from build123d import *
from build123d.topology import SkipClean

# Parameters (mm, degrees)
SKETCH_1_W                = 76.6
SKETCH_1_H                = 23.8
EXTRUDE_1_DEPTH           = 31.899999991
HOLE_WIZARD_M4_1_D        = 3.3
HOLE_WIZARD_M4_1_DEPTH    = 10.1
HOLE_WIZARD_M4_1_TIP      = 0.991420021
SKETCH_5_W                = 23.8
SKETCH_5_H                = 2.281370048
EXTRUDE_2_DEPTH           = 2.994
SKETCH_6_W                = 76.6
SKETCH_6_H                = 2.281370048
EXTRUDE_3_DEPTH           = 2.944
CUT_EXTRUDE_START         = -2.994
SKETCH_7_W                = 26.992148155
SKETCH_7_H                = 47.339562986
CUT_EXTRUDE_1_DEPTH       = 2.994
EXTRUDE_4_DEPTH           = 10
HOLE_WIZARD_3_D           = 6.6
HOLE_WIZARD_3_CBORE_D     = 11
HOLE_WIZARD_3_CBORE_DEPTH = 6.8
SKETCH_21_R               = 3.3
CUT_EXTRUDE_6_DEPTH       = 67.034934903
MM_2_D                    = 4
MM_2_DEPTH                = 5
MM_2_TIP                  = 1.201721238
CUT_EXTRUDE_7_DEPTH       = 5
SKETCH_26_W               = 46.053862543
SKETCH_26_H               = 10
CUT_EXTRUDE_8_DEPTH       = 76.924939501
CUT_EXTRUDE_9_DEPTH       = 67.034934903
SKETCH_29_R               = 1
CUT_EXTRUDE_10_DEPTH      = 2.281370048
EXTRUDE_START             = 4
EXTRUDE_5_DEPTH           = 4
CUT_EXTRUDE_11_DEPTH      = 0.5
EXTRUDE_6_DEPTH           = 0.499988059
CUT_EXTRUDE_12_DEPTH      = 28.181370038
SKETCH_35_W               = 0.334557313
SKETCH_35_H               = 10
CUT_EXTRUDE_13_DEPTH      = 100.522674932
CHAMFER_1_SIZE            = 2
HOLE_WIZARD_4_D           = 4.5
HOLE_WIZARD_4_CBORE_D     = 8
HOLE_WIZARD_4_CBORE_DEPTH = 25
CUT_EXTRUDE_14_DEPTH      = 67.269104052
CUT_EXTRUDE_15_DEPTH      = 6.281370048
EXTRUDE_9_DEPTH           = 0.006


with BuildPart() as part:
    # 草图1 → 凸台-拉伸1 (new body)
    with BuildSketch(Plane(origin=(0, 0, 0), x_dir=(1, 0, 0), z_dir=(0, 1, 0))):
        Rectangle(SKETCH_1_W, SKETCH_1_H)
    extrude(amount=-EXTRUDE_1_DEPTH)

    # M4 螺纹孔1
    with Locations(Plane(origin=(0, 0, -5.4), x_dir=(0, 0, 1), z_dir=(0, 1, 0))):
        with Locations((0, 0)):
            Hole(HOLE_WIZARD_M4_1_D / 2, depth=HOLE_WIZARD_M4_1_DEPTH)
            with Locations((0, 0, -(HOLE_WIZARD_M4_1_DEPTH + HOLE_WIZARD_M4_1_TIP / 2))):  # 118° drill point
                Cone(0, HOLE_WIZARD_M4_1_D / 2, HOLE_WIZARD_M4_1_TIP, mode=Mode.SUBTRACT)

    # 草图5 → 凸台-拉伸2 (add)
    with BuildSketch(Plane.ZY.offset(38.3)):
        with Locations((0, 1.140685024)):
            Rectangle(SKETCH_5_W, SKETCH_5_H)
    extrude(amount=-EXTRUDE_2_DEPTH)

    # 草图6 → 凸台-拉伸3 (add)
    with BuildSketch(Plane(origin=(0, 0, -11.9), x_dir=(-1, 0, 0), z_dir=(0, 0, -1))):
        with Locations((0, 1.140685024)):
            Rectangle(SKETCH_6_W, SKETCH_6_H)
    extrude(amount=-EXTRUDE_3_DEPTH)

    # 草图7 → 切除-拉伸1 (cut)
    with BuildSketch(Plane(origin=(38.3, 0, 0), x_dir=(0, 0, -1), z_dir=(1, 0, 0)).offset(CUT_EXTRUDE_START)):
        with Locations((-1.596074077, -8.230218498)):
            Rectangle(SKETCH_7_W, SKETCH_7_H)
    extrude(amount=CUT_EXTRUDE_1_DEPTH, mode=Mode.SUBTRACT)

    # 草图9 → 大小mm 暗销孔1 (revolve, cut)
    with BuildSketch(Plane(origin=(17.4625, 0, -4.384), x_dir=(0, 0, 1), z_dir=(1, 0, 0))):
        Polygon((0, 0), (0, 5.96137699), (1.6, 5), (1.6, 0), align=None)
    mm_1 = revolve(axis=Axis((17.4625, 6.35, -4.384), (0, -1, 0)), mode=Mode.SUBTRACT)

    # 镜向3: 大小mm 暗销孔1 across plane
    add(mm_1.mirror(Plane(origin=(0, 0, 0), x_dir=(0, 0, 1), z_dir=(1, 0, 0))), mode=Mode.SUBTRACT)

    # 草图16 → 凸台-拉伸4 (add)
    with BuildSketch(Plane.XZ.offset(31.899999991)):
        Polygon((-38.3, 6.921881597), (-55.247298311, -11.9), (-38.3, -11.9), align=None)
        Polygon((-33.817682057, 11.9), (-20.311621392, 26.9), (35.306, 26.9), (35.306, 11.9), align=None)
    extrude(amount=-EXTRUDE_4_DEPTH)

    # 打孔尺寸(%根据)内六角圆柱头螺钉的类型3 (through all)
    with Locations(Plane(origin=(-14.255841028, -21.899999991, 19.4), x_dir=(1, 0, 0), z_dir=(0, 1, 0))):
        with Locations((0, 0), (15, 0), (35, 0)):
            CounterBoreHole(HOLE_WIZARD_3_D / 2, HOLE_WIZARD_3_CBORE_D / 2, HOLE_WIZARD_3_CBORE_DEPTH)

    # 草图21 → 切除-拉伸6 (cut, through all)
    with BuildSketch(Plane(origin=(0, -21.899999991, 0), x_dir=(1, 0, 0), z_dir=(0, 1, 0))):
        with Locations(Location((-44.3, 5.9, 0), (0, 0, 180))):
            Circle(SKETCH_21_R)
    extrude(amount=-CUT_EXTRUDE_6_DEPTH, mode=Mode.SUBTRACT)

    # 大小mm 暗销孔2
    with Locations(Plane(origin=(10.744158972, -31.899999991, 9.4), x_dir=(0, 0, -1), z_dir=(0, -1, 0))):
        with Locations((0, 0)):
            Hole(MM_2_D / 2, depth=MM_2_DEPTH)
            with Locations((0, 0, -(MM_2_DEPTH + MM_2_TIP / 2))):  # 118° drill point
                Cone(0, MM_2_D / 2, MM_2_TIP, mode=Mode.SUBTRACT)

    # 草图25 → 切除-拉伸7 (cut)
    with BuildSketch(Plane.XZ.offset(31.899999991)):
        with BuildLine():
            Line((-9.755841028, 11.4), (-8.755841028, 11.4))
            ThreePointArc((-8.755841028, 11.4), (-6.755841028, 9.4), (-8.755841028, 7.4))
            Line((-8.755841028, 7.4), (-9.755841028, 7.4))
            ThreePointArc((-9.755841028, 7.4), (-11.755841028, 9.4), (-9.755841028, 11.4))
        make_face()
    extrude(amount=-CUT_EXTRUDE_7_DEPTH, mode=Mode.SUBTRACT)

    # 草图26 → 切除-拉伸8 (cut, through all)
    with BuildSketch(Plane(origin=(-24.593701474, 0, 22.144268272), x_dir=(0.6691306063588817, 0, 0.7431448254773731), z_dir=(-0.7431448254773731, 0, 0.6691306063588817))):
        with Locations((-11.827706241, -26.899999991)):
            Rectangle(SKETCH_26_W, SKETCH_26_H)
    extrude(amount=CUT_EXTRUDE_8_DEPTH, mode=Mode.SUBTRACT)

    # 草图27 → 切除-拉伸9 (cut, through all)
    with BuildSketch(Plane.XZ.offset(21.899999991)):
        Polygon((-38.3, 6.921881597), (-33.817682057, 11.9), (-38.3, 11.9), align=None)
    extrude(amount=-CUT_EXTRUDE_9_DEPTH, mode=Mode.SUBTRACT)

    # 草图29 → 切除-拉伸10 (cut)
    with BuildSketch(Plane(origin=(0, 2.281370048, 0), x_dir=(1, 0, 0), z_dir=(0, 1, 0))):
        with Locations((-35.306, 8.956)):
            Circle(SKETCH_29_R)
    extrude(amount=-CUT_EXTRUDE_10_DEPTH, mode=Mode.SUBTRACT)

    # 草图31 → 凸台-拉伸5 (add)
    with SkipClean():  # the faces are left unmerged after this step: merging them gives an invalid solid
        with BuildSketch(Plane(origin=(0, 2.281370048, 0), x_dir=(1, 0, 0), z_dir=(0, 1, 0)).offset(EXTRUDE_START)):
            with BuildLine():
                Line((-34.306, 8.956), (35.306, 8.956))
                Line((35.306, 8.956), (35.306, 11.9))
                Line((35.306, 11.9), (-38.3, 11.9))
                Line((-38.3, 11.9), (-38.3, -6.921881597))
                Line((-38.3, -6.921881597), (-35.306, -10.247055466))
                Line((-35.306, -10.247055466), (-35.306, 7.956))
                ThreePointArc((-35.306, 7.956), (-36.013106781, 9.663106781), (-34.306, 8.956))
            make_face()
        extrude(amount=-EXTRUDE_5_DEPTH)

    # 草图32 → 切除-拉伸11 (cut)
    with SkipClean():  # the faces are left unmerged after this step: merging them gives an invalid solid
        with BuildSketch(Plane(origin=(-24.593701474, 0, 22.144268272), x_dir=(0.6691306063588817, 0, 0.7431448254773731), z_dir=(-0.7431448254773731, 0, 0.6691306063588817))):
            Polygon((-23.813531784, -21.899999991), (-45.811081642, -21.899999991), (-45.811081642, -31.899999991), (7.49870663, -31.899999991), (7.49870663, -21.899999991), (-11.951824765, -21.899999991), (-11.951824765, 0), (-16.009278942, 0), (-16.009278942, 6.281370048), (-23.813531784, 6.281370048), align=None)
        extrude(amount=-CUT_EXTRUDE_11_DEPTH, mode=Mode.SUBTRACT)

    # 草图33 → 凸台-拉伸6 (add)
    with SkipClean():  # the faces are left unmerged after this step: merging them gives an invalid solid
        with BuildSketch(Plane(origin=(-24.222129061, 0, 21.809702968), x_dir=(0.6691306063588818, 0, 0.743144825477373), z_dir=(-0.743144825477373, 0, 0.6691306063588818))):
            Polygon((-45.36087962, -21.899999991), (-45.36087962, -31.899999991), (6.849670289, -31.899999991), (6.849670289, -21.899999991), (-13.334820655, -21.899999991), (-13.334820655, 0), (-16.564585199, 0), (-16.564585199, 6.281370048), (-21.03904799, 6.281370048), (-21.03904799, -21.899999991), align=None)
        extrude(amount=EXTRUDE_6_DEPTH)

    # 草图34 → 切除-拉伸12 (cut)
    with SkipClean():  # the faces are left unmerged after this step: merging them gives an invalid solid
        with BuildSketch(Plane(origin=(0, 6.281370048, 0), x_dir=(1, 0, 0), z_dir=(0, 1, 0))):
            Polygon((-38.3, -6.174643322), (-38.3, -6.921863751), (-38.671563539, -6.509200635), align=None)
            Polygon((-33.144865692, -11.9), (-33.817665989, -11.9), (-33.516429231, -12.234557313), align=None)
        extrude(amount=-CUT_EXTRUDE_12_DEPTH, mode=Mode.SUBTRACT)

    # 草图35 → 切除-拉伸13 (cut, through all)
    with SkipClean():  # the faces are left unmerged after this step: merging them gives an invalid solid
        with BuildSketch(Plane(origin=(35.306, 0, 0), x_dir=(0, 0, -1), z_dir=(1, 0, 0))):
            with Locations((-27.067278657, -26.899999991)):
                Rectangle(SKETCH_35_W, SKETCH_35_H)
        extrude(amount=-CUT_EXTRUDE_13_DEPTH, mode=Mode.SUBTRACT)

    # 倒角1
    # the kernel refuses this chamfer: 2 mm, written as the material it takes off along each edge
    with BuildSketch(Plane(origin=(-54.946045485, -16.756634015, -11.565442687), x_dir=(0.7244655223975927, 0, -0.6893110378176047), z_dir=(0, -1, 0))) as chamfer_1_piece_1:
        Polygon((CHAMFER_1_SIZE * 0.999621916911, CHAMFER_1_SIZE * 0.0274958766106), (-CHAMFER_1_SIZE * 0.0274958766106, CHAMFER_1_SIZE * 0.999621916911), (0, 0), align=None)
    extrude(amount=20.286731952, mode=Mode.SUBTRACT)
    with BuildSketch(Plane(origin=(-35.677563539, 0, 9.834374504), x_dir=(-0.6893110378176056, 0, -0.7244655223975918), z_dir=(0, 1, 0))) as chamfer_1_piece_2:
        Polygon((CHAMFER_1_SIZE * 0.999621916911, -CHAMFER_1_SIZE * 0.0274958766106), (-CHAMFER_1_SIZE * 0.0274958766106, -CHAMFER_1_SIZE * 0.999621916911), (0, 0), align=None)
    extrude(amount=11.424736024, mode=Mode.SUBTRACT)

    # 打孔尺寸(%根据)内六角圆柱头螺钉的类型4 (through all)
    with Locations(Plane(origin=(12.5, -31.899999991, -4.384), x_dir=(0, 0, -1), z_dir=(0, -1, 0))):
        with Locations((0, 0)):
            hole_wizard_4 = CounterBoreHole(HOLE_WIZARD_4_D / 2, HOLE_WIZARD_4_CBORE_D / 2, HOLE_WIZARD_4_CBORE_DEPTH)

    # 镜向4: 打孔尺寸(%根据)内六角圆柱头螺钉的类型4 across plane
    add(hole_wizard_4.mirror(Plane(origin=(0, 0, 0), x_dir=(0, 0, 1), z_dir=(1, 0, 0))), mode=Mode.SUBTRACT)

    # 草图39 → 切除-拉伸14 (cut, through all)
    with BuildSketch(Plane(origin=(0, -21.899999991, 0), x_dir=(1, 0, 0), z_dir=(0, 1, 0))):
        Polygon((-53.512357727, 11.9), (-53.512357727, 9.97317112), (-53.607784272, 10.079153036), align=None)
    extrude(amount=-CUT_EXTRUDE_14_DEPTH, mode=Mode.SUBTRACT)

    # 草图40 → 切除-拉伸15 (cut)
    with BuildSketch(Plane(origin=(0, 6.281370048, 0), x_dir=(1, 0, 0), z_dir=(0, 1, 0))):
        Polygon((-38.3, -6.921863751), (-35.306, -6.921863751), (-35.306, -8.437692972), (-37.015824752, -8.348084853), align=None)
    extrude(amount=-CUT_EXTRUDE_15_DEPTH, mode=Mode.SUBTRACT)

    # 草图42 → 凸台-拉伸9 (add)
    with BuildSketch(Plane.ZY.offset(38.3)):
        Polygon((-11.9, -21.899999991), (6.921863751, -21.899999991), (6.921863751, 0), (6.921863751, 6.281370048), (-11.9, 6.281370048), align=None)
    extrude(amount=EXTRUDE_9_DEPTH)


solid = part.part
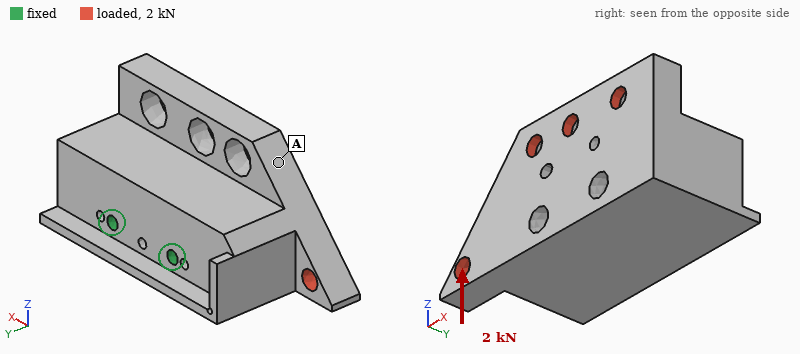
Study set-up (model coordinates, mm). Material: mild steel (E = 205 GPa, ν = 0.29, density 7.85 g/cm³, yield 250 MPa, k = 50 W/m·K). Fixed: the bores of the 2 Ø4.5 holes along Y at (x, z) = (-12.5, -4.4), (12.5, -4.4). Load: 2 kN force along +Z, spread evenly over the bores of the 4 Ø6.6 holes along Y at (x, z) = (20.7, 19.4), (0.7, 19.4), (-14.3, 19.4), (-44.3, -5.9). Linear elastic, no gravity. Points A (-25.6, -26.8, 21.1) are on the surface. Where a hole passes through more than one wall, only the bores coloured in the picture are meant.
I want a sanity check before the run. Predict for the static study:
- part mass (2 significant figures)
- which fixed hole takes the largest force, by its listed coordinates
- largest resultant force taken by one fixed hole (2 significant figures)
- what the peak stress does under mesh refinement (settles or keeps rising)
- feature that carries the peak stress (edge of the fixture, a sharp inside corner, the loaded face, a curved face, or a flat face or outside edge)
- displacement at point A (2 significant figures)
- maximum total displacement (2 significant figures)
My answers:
490 g
(-12.5, -4.4)
2.5 kN
keeps rising
edge of the fixture
27 µm
32 µm
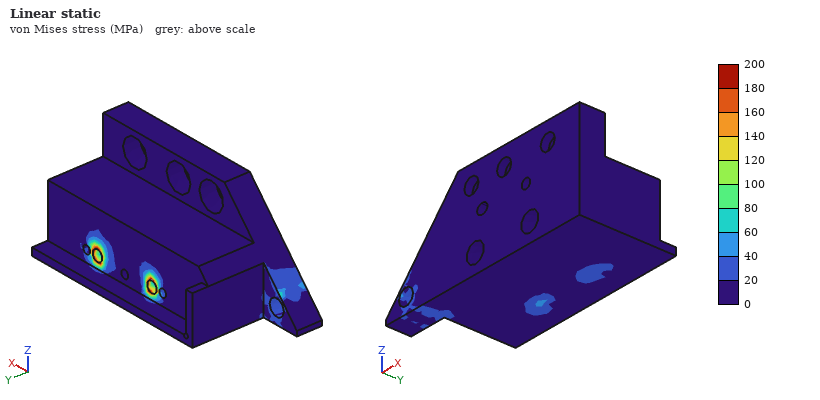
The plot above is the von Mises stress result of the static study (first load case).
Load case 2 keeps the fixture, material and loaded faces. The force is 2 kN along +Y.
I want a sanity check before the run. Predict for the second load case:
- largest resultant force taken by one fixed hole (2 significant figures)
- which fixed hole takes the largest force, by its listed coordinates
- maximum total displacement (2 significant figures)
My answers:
2.5 kN
(-12.5, -4.4)
16 µm
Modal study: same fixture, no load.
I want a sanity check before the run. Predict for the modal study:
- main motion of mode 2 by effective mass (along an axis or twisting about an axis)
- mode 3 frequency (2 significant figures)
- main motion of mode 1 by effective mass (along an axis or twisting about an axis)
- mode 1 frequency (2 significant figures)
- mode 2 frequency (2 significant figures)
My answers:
along X
6200 Hz
along Z
3100 Hz
5900 Hz
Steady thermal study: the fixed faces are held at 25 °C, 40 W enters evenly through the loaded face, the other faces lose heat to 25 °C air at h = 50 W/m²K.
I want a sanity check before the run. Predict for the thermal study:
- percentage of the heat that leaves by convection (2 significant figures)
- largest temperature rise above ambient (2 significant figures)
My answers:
32 %
74 K
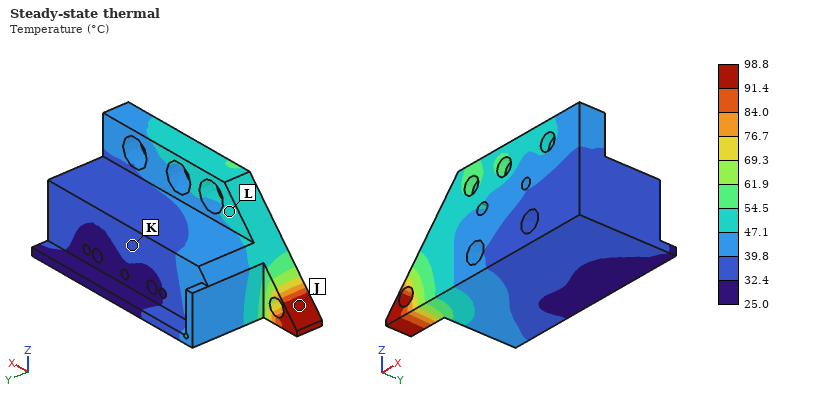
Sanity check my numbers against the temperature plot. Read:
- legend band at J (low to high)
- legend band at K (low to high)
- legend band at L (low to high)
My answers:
91.4 to 98.8 °C
32.4 to 39.8 °C
47.1 to 54.5 °C
